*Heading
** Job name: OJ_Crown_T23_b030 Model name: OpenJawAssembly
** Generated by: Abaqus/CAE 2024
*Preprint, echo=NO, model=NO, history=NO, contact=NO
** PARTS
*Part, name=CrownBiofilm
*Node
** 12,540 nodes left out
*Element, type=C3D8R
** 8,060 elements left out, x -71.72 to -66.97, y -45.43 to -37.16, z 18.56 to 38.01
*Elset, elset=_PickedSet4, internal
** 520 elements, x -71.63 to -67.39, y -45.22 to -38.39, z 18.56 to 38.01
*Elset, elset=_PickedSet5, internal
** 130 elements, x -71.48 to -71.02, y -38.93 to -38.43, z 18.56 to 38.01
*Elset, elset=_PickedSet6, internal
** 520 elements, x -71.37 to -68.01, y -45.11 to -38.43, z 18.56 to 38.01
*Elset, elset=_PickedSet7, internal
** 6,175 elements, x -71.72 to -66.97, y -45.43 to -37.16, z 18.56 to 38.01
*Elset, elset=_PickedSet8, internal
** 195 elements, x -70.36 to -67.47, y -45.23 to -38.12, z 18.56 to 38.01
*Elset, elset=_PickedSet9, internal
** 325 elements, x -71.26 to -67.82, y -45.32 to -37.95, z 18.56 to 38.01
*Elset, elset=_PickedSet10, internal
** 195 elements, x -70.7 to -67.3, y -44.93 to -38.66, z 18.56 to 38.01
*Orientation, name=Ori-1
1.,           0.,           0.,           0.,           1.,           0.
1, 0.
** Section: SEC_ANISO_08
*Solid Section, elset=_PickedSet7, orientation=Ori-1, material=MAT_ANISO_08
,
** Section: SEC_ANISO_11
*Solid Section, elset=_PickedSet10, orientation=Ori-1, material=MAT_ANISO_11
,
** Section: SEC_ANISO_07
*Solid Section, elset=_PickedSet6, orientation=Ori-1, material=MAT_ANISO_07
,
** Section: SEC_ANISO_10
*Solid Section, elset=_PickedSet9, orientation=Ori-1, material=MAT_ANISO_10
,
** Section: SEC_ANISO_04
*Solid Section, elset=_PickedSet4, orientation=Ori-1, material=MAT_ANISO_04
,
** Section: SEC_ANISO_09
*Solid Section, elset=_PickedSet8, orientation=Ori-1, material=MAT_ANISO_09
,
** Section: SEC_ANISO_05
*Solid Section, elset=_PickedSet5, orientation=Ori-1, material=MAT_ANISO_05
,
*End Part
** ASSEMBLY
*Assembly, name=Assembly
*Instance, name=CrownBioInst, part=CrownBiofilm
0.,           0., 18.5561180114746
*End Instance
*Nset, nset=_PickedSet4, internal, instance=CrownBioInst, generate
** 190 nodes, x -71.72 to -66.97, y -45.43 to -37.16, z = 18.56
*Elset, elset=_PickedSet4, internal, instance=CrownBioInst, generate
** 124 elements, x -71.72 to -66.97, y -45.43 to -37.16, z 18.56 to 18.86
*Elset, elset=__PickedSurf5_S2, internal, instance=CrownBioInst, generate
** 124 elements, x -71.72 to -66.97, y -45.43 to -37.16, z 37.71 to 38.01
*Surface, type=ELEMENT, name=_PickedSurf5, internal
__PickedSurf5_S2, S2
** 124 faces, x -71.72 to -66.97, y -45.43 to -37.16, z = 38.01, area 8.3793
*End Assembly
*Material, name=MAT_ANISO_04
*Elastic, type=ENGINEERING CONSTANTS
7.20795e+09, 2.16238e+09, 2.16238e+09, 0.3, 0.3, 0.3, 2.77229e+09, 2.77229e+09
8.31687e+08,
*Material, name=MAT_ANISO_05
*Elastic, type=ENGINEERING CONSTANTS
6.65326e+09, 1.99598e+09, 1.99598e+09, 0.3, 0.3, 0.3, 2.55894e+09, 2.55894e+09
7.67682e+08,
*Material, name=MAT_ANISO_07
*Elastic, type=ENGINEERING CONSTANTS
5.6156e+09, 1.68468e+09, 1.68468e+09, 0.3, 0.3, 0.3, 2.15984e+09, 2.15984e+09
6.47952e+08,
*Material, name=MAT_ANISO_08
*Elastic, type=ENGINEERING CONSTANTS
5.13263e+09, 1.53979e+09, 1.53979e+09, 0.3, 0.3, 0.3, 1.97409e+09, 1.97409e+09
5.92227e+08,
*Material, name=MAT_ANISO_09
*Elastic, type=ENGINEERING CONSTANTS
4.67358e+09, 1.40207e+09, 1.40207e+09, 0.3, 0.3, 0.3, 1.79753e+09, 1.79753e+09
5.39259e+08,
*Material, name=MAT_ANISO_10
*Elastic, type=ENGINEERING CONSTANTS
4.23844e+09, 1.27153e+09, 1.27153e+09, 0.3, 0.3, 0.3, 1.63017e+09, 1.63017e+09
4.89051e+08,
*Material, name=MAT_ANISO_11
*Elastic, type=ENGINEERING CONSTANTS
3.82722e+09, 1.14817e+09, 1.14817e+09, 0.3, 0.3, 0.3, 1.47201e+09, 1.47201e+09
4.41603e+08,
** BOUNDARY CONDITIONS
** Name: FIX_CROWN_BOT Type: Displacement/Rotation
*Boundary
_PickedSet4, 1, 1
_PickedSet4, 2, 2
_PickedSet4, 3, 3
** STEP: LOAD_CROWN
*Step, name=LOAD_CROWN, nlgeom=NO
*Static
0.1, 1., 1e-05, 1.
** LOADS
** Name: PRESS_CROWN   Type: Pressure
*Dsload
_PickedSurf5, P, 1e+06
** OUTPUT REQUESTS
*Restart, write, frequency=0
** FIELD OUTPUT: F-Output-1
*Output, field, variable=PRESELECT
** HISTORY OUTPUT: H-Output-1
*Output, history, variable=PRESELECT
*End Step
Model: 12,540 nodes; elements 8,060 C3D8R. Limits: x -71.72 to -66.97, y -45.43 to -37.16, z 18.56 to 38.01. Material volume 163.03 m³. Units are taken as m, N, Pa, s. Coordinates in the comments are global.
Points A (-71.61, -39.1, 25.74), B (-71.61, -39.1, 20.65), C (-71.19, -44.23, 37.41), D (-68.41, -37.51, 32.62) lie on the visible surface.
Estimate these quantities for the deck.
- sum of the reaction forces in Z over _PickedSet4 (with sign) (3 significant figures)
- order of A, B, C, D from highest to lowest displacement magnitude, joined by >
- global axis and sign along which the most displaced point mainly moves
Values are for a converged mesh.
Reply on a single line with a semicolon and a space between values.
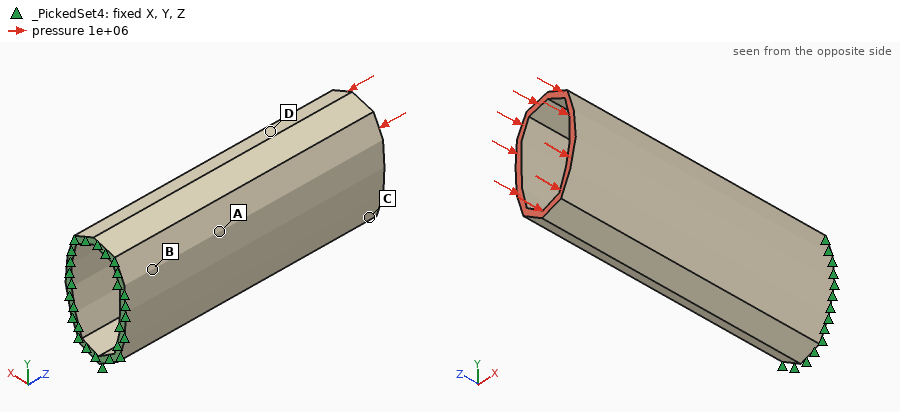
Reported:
8.38e+06 N; C > D > A > B; -Z
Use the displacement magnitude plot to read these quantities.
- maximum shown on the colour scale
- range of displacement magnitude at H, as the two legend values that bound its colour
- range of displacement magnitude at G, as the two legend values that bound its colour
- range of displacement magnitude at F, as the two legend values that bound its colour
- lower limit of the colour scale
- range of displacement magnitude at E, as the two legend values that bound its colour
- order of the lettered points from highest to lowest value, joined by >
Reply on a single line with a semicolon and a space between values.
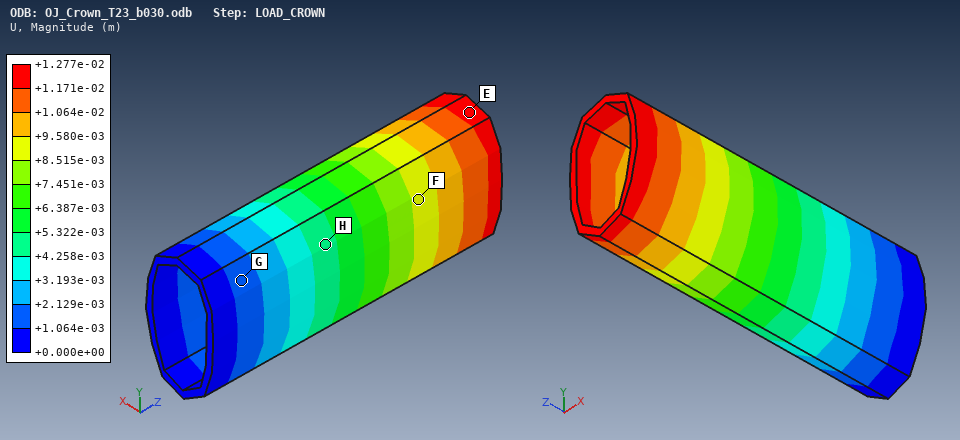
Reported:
+1.277e-02 m; +4.258e-03 to +5.322e-03 m; +1.064e-03 to +2.129e-03 m; +8.515e-03 to +9.580e-03 m; +0.000e+00 m; +1.171e-02 to +1.277e-02 m; E > F > H > G
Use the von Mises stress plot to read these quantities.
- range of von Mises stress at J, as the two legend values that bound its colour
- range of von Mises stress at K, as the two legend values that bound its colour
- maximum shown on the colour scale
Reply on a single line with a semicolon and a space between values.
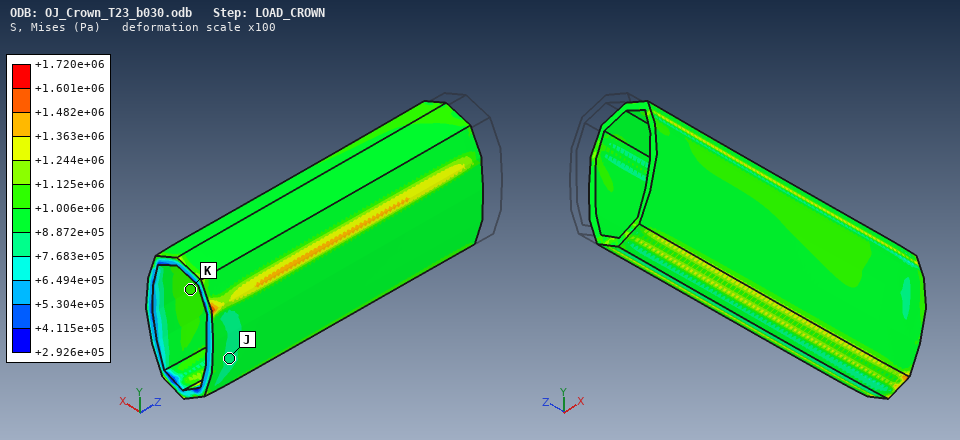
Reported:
+7.683e+05 to +8.872e+05 Pa; +1.006e+06 to +1.125e+06 Pa; +1.720e+06 Pa
